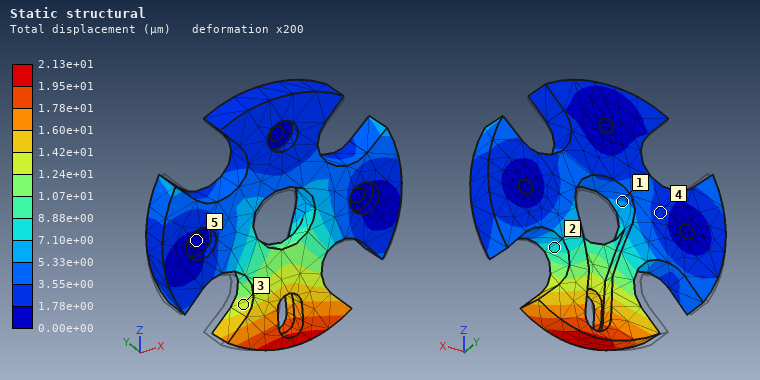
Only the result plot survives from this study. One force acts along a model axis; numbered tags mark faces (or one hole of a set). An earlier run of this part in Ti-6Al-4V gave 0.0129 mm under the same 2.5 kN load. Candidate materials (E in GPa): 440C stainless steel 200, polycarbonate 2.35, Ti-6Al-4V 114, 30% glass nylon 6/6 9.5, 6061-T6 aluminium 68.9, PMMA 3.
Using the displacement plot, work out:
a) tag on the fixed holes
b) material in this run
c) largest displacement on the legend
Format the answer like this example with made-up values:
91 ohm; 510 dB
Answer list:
5; 6061-T6 aluminium; 2.13e+01 µm
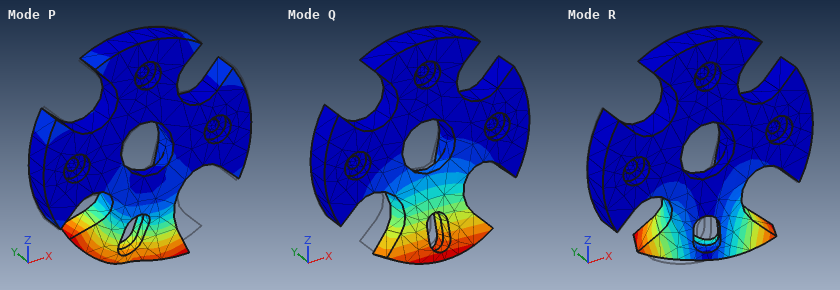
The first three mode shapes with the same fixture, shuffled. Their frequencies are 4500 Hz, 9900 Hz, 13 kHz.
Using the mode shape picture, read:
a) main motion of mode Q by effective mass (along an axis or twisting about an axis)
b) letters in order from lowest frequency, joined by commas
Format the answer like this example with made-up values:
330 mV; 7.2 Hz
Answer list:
along Y; Q, R, P
